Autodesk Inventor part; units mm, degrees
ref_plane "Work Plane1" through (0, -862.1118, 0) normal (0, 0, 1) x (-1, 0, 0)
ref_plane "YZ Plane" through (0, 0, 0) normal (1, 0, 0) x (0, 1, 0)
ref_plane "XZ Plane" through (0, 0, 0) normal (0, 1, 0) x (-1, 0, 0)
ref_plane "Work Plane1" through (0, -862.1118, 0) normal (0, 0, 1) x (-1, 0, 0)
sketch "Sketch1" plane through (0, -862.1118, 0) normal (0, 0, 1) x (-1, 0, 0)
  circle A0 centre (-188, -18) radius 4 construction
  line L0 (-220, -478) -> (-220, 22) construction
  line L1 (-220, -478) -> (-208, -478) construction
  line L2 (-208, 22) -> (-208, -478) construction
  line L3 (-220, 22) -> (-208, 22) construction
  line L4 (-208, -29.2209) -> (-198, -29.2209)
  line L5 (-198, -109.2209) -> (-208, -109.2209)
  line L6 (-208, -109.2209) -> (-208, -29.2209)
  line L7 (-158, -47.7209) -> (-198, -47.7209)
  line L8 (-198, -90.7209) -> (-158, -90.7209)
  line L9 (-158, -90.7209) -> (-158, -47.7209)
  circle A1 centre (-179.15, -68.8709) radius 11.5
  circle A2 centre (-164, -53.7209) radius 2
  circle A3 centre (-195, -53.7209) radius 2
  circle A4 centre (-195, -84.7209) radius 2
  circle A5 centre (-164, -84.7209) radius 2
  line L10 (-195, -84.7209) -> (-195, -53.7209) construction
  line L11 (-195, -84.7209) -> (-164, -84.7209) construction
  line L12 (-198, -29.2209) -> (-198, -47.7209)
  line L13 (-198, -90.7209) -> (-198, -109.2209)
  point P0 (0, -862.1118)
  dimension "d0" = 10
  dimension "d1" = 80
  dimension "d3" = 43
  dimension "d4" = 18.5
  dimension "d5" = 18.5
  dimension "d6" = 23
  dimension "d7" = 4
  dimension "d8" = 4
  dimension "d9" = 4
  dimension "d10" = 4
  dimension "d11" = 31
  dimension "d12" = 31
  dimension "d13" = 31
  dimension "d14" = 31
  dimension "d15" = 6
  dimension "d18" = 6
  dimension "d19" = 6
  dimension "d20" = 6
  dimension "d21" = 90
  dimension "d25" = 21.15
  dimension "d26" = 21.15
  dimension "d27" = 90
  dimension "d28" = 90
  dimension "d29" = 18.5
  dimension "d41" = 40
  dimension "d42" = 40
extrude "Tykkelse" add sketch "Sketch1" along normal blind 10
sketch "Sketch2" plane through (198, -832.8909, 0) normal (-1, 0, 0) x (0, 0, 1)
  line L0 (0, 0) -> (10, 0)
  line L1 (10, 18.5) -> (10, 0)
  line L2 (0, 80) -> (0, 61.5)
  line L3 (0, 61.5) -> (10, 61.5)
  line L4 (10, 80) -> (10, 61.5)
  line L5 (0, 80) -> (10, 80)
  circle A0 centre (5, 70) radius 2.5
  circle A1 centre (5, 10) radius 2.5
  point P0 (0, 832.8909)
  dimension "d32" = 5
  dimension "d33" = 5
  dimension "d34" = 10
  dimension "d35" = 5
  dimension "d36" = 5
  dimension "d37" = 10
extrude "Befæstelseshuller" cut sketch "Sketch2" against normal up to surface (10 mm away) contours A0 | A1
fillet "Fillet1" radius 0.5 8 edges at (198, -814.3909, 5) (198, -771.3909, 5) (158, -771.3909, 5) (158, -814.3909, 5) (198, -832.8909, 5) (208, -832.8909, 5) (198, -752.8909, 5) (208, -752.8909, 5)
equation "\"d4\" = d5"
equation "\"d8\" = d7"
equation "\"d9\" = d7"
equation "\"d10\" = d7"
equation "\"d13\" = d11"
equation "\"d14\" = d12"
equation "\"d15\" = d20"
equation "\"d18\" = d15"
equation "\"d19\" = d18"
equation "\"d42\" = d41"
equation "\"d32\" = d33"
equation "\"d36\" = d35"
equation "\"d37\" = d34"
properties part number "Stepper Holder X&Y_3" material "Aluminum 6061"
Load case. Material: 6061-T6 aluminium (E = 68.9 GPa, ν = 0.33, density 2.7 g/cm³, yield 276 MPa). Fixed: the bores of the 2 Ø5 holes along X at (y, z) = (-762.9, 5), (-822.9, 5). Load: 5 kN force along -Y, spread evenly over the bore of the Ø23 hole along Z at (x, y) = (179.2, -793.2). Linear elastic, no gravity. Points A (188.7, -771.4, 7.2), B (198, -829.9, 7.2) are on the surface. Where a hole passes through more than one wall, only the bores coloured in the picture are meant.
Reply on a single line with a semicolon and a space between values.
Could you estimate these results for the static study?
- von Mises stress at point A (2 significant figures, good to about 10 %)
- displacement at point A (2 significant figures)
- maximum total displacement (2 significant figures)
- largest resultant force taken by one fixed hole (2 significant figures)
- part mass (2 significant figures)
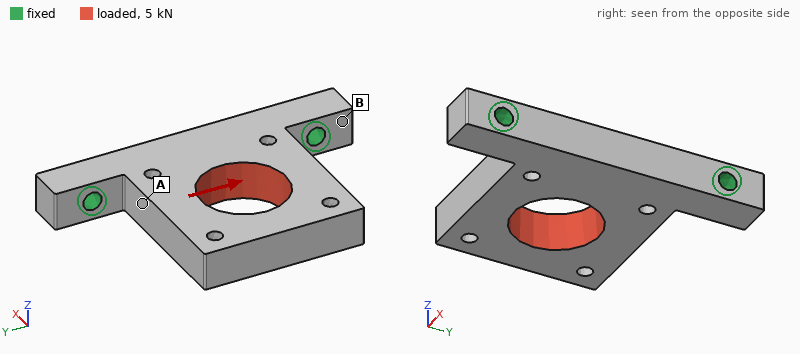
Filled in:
45 MPa; 30 µm; 81 µm; 3.5 kN; 54 g
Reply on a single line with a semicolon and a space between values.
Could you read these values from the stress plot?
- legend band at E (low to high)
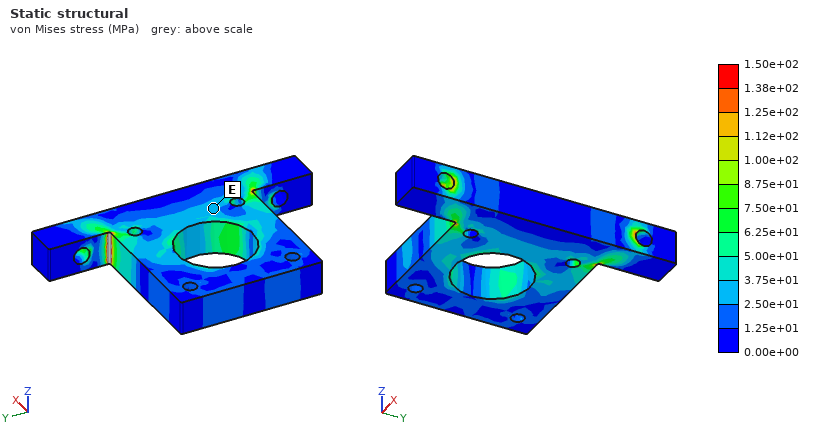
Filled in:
2.50e+01 to 3.75e+01 MPa
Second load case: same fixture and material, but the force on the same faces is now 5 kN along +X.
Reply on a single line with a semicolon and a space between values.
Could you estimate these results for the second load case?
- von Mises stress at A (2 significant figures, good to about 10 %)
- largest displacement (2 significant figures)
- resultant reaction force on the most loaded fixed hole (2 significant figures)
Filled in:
25 MPa; 29 µm; 2.7 kN
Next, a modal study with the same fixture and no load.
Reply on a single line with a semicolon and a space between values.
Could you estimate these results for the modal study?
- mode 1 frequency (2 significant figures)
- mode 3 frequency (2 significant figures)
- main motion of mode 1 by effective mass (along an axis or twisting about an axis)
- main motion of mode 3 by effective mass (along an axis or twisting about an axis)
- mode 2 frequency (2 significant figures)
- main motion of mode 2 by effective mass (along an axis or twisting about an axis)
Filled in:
2100 Hz; 7300 Hz; along Z; along Y; 6500 Hz; twisting about X
